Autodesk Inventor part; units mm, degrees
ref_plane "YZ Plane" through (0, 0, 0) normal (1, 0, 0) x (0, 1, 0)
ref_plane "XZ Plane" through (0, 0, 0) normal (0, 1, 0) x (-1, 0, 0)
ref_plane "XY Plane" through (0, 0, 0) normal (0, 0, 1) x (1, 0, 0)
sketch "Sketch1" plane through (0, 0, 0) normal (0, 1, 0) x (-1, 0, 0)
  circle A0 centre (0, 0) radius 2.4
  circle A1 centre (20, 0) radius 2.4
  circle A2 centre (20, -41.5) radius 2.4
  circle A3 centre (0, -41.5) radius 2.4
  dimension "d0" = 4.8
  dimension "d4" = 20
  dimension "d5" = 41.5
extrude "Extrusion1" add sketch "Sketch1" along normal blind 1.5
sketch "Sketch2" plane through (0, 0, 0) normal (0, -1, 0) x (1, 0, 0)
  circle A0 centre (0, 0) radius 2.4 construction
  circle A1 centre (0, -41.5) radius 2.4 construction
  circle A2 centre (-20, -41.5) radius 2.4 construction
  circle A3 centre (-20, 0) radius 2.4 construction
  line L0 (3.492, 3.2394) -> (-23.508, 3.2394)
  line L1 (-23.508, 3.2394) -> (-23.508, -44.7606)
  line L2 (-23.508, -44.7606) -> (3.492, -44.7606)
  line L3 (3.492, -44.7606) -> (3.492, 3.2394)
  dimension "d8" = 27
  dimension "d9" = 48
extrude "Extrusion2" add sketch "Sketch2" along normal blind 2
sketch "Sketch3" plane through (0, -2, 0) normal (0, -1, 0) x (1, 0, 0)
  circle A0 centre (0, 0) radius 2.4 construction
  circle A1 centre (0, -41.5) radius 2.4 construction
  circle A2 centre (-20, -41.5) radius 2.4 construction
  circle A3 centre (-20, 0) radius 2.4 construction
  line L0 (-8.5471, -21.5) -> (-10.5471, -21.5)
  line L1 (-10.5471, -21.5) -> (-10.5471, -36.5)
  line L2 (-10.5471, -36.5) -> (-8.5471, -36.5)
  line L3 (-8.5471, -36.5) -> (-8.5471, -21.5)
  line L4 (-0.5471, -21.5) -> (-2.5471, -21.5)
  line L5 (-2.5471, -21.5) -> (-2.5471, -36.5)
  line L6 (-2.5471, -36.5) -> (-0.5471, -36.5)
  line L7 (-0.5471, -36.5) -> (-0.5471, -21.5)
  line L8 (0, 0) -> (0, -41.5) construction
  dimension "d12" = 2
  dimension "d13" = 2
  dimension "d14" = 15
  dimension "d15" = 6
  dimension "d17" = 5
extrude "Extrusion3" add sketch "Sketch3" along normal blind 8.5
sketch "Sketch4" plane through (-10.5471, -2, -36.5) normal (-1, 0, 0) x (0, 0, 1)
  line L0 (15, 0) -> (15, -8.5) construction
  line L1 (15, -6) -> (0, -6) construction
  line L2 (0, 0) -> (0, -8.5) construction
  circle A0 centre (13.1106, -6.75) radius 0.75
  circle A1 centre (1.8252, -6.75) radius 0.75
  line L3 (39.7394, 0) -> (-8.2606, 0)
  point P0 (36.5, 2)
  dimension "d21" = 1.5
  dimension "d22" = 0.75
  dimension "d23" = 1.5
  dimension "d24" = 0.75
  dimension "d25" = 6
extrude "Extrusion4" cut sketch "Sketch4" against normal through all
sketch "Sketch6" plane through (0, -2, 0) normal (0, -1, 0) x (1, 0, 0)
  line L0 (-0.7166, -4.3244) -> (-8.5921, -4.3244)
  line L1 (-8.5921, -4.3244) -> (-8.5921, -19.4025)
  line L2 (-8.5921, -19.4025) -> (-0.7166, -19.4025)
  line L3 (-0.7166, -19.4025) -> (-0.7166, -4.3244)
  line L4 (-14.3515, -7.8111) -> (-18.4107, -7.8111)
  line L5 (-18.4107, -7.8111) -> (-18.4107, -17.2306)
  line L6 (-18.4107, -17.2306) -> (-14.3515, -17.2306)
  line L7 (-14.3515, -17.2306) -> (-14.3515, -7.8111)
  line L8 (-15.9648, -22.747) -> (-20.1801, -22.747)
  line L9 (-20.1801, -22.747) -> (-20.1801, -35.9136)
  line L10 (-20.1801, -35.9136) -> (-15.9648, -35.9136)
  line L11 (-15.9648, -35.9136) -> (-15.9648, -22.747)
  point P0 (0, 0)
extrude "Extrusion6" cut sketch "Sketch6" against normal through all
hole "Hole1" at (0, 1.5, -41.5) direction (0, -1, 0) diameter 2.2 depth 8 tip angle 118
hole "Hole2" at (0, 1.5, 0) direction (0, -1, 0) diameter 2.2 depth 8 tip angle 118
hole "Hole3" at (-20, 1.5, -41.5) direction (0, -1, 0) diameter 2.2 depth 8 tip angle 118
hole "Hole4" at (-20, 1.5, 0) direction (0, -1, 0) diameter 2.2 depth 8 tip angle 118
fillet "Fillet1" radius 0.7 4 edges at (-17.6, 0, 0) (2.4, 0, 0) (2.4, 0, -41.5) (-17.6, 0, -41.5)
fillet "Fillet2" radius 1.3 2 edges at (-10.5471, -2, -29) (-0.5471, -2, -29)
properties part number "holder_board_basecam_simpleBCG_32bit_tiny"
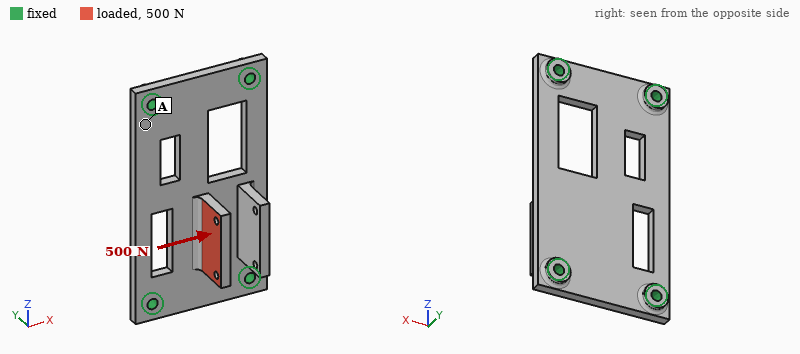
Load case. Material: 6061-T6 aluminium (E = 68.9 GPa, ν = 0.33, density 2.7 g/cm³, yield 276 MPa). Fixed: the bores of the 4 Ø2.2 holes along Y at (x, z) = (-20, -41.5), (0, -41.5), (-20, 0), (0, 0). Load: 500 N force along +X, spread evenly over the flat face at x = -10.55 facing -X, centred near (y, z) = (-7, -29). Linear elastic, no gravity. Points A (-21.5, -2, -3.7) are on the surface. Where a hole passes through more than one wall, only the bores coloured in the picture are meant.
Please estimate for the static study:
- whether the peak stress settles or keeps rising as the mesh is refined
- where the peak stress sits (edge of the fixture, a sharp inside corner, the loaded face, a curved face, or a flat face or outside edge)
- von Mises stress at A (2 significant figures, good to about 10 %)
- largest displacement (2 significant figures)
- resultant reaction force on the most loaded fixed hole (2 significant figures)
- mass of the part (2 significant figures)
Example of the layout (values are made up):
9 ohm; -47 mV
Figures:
keeps rising; a sharp inside corner; 25 MPa; 0.15 mm; 340 N; 7.4 g
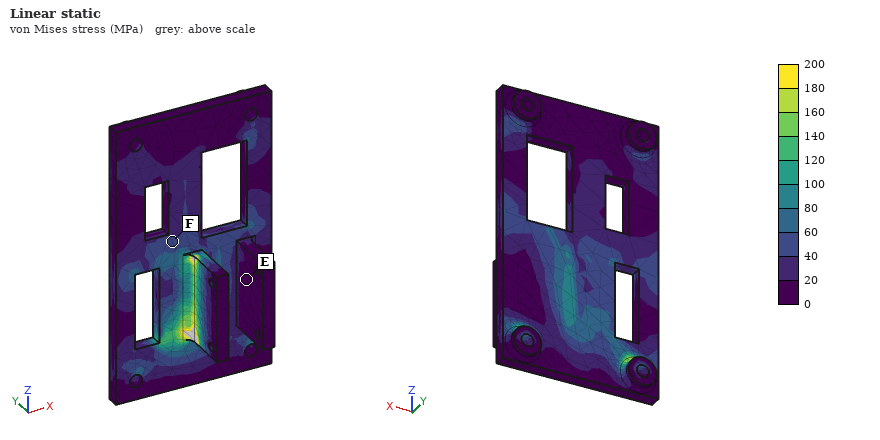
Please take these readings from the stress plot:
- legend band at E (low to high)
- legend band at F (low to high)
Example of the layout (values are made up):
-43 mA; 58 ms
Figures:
0 to 20 MPa; 40 to 60 MPa
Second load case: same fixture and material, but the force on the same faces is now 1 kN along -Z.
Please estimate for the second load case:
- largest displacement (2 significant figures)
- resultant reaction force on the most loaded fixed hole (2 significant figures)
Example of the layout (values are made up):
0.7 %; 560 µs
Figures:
0.19 mm; 390 N
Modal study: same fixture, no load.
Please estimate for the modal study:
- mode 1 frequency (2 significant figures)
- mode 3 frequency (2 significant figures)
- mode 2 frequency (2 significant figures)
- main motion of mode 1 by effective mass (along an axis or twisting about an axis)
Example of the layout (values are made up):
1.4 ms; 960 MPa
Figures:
5300 Hz; 12 kHz; 8000 Hz; along Y
